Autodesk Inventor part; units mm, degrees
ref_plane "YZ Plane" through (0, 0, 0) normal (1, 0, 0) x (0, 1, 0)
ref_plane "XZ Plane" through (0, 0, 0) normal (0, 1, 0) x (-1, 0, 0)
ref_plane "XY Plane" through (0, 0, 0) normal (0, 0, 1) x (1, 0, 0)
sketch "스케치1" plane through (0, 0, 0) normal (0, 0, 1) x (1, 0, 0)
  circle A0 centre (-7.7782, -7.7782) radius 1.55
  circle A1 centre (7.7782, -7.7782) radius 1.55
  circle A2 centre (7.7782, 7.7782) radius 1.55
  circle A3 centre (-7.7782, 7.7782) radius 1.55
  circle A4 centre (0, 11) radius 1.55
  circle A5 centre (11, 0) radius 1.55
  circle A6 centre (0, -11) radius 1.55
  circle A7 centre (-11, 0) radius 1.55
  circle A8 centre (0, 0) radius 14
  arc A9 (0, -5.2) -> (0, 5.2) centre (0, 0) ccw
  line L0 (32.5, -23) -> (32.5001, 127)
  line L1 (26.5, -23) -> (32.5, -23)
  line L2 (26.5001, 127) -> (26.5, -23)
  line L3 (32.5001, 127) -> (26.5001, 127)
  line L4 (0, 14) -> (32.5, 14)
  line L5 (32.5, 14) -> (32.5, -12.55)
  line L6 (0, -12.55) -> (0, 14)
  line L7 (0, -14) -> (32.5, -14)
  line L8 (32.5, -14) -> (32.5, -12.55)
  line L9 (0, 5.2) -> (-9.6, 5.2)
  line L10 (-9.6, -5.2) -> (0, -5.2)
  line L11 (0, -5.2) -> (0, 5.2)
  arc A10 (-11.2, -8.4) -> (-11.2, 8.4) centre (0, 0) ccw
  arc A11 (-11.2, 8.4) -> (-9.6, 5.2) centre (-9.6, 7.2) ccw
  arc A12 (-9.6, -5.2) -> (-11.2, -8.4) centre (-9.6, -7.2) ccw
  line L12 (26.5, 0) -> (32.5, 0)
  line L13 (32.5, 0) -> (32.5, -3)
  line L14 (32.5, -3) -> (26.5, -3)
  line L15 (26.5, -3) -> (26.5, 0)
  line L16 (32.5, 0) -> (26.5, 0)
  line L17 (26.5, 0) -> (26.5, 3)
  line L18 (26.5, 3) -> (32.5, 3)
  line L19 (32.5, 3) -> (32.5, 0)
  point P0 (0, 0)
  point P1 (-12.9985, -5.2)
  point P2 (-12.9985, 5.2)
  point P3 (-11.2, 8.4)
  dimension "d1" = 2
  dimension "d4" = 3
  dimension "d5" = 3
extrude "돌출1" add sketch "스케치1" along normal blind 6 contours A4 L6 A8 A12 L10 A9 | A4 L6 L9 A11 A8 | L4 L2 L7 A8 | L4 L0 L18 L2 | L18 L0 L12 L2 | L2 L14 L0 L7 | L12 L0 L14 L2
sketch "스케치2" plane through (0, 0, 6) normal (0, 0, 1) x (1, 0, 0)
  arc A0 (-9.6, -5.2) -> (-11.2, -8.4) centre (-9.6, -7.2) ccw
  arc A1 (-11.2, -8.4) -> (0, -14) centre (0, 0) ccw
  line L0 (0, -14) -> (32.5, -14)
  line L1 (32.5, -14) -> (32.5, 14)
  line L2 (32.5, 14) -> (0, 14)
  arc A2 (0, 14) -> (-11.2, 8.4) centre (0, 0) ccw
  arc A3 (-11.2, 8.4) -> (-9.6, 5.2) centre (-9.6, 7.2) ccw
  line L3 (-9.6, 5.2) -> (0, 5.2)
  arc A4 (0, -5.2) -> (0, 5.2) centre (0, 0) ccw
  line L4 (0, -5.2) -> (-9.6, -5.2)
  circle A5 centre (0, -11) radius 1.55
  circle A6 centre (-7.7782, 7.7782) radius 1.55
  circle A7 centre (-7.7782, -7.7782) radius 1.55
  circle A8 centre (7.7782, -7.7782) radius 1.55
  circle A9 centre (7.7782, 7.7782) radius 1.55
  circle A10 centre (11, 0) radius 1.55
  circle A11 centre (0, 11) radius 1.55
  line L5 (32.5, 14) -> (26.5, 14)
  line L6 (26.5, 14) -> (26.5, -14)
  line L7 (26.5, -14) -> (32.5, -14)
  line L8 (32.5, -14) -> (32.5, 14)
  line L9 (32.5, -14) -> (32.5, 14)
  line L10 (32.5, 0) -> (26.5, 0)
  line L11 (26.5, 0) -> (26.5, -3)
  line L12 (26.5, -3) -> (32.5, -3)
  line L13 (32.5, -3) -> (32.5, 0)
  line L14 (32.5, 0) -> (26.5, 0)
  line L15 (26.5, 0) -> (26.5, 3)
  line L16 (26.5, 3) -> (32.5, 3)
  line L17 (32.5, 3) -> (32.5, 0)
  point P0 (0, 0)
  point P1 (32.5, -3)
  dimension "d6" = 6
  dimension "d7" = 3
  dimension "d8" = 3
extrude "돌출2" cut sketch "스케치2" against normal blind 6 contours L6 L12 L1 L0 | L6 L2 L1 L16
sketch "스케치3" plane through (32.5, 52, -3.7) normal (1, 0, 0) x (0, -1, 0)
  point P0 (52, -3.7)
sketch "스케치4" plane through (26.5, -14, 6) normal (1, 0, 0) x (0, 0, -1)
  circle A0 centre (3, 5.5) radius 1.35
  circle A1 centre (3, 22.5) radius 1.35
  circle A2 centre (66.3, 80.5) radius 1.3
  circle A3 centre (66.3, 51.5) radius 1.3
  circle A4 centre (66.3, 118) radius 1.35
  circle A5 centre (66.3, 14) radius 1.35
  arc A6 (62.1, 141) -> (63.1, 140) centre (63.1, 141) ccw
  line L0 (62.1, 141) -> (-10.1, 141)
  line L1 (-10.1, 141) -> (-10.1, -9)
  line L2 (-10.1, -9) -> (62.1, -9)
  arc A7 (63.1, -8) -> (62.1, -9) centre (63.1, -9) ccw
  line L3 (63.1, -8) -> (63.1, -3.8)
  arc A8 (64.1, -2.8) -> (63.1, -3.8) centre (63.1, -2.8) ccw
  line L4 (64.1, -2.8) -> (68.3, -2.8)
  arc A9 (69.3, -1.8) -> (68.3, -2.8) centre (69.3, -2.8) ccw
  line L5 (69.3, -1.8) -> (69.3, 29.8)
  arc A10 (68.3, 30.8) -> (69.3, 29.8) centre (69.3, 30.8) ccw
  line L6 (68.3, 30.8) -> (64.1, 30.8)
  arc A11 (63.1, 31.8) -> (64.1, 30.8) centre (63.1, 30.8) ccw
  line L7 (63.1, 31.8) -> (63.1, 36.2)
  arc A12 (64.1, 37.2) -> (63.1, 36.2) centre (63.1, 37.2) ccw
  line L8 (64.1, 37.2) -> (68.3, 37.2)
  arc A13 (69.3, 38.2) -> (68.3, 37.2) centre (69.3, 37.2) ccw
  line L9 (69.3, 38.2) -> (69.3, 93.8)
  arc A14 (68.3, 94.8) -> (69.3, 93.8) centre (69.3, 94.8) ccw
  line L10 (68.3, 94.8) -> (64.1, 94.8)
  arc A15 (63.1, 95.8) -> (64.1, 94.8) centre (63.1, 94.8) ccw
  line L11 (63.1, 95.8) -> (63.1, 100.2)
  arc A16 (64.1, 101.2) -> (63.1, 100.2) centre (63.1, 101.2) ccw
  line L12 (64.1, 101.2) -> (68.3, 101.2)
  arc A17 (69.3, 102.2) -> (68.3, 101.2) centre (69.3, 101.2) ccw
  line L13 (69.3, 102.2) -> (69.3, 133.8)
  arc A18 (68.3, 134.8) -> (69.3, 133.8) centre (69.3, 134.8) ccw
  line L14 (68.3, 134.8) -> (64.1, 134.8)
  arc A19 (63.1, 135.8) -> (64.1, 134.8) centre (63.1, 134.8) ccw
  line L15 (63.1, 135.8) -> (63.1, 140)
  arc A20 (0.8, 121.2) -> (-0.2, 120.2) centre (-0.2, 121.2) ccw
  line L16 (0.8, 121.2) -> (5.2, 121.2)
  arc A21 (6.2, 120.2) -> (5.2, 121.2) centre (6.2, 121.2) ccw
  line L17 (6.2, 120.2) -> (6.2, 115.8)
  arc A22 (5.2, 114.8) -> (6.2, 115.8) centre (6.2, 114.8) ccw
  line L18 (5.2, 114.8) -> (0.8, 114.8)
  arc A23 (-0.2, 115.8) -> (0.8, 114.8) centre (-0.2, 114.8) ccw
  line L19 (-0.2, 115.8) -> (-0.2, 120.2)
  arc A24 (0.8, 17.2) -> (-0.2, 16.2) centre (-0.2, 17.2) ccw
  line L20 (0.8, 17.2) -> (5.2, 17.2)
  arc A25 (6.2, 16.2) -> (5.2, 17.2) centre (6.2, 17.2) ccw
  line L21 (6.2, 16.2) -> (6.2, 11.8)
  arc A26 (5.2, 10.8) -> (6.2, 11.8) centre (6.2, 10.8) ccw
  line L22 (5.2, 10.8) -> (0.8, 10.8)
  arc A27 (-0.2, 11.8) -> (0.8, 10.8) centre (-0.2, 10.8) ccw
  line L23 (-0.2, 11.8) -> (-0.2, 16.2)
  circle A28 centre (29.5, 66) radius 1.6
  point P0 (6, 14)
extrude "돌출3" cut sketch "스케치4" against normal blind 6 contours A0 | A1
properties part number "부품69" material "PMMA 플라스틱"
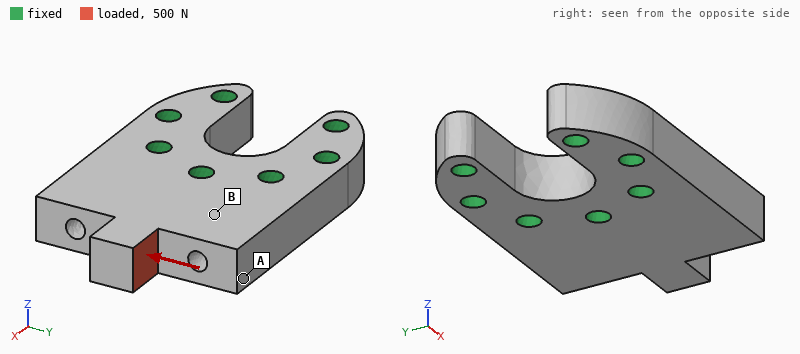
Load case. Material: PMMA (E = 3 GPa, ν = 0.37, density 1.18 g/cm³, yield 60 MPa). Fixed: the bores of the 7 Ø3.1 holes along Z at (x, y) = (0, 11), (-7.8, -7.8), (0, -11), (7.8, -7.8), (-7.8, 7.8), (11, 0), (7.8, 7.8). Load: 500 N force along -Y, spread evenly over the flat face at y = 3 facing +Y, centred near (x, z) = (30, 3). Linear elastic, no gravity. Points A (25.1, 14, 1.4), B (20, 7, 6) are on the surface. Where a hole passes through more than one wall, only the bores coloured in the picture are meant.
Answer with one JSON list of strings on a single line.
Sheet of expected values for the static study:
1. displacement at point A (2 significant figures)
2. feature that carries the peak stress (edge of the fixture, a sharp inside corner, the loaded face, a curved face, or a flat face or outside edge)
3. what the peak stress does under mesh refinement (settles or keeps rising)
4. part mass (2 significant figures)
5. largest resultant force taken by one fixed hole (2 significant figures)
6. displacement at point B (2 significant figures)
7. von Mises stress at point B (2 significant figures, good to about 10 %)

["0.096 mm", "a sharp inside corner", "keeps rising", "5.9 g", "380 N", "0.062 mm", "11 MPa"]
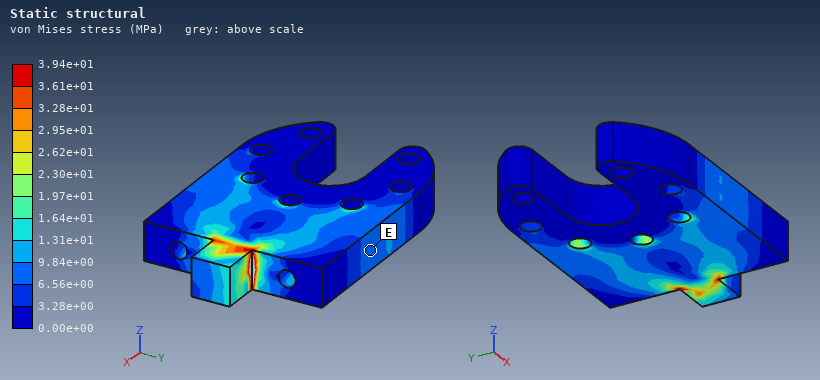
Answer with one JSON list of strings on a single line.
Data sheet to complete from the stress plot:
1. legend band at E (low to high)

["6.56e+00 to 9.84e+00 MPa"]
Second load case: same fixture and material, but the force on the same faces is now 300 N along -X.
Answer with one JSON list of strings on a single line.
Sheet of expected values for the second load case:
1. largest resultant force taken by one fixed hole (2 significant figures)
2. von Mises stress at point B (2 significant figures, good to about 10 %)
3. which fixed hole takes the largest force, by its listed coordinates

["130 N", "3.6 MPa", "(11, 0)"]
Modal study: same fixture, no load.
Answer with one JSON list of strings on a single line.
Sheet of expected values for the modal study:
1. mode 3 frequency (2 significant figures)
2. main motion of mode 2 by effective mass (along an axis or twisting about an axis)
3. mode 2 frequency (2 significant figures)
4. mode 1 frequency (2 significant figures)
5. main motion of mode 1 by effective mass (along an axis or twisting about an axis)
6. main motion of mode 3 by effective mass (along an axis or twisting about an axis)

["9300 Hz", "twisting about X", "7000 Hz", "4300 Hz", "along Z", "along Y"]
